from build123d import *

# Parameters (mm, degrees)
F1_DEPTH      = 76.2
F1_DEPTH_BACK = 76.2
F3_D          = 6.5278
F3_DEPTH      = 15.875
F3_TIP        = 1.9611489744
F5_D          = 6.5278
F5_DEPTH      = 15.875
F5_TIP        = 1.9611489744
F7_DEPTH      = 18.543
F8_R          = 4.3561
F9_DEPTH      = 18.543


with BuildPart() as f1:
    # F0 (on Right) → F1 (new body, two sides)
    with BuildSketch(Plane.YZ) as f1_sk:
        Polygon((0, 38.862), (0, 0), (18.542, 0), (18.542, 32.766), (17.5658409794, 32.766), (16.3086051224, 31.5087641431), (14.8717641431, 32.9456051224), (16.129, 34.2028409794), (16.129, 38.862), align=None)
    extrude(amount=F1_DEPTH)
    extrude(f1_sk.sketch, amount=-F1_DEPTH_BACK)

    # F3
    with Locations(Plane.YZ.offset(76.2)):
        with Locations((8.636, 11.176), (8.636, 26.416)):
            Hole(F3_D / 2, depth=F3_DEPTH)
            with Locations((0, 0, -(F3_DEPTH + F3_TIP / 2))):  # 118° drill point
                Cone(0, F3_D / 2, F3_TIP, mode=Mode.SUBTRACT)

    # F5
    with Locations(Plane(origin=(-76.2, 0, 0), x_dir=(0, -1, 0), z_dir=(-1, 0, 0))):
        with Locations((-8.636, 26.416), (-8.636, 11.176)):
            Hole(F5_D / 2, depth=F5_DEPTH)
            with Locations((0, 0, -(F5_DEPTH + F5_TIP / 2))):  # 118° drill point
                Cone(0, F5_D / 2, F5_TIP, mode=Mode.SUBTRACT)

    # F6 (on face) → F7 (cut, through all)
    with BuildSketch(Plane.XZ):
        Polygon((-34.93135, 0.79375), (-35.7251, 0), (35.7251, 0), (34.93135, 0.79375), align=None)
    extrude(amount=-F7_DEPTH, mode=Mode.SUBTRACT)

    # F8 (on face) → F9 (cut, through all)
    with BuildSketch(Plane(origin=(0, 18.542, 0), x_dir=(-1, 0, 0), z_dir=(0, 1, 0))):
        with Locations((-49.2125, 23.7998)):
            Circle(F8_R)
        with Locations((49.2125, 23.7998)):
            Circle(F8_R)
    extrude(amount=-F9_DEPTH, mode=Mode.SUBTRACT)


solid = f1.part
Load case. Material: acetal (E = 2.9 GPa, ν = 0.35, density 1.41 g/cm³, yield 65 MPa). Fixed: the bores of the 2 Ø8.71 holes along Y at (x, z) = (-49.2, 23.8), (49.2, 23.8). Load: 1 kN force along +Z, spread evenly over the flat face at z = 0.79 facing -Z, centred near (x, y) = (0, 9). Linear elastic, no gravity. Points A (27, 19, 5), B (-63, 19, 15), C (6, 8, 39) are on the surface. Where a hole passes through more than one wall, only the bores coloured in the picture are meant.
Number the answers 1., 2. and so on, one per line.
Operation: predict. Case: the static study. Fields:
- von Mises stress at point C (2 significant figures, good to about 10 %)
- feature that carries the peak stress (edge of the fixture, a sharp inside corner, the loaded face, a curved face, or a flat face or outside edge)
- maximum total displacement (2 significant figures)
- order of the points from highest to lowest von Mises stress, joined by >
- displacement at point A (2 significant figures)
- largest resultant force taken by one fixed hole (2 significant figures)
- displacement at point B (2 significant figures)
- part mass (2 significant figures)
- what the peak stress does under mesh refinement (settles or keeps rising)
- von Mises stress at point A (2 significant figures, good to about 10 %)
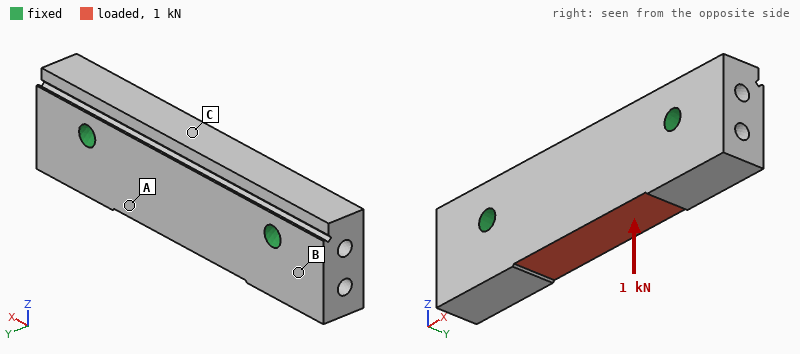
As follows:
1. 2.2 MPa
2. edge of the fixture
3. 58 µm
4. C > A > B
5. 39 µm
6. 550 N
7. 11 µm
8. 140 g
9. keeps rising
10. 1.2 MPa
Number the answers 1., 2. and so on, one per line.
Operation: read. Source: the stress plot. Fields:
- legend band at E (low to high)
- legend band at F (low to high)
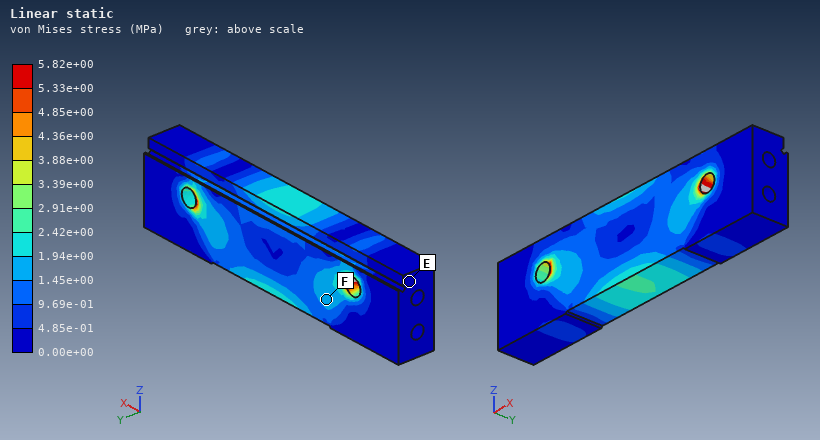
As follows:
1. 0.00e+00 to 4.85e-01 MPa
2. 1.45e+00 to 1.94e+00 MPa
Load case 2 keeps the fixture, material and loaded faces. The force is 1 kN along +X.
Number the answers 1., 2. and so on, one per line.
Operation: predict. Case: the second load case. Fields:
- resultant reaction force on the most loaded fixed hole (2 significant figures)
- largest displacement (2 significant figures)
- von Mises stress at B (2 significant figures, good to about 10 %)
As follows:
1. 550 N
2. 19 µm
3. 0.25 MPa
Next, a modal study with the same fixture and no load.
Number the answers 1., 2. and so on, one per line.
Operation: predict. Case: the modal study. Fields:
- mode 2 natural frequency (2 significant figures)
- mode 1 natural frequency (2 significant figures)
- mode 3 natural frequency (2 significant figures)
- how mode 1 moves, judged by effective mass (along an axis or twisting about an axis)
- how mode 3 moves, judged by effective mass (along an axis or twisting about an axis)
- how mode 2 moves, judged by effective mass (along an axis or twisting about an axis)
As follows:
1. 2500 Hz
2. 2200 Hz
3. 3100 Hz
4. along Y
5. twisting about X
6. along Z
